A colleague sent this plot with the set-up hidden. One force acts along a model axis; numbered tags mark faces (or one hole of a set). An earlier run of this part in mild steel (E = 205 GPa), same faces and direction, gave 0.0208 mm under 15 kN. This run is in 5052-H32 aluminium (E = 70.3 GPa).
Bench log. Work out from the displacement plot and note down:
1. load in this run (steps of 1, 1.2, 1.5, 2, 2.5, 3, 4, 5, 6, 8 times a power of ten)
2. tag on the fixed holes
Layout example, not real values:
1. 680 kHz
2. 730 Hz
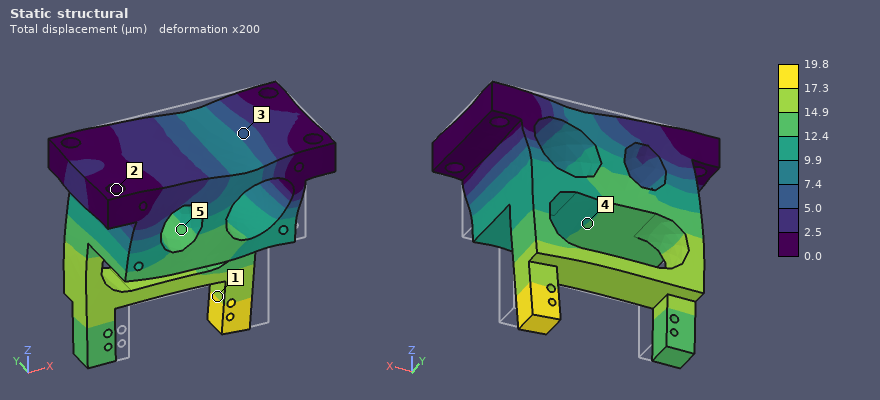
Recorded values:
1. 5 kN
2. 2
